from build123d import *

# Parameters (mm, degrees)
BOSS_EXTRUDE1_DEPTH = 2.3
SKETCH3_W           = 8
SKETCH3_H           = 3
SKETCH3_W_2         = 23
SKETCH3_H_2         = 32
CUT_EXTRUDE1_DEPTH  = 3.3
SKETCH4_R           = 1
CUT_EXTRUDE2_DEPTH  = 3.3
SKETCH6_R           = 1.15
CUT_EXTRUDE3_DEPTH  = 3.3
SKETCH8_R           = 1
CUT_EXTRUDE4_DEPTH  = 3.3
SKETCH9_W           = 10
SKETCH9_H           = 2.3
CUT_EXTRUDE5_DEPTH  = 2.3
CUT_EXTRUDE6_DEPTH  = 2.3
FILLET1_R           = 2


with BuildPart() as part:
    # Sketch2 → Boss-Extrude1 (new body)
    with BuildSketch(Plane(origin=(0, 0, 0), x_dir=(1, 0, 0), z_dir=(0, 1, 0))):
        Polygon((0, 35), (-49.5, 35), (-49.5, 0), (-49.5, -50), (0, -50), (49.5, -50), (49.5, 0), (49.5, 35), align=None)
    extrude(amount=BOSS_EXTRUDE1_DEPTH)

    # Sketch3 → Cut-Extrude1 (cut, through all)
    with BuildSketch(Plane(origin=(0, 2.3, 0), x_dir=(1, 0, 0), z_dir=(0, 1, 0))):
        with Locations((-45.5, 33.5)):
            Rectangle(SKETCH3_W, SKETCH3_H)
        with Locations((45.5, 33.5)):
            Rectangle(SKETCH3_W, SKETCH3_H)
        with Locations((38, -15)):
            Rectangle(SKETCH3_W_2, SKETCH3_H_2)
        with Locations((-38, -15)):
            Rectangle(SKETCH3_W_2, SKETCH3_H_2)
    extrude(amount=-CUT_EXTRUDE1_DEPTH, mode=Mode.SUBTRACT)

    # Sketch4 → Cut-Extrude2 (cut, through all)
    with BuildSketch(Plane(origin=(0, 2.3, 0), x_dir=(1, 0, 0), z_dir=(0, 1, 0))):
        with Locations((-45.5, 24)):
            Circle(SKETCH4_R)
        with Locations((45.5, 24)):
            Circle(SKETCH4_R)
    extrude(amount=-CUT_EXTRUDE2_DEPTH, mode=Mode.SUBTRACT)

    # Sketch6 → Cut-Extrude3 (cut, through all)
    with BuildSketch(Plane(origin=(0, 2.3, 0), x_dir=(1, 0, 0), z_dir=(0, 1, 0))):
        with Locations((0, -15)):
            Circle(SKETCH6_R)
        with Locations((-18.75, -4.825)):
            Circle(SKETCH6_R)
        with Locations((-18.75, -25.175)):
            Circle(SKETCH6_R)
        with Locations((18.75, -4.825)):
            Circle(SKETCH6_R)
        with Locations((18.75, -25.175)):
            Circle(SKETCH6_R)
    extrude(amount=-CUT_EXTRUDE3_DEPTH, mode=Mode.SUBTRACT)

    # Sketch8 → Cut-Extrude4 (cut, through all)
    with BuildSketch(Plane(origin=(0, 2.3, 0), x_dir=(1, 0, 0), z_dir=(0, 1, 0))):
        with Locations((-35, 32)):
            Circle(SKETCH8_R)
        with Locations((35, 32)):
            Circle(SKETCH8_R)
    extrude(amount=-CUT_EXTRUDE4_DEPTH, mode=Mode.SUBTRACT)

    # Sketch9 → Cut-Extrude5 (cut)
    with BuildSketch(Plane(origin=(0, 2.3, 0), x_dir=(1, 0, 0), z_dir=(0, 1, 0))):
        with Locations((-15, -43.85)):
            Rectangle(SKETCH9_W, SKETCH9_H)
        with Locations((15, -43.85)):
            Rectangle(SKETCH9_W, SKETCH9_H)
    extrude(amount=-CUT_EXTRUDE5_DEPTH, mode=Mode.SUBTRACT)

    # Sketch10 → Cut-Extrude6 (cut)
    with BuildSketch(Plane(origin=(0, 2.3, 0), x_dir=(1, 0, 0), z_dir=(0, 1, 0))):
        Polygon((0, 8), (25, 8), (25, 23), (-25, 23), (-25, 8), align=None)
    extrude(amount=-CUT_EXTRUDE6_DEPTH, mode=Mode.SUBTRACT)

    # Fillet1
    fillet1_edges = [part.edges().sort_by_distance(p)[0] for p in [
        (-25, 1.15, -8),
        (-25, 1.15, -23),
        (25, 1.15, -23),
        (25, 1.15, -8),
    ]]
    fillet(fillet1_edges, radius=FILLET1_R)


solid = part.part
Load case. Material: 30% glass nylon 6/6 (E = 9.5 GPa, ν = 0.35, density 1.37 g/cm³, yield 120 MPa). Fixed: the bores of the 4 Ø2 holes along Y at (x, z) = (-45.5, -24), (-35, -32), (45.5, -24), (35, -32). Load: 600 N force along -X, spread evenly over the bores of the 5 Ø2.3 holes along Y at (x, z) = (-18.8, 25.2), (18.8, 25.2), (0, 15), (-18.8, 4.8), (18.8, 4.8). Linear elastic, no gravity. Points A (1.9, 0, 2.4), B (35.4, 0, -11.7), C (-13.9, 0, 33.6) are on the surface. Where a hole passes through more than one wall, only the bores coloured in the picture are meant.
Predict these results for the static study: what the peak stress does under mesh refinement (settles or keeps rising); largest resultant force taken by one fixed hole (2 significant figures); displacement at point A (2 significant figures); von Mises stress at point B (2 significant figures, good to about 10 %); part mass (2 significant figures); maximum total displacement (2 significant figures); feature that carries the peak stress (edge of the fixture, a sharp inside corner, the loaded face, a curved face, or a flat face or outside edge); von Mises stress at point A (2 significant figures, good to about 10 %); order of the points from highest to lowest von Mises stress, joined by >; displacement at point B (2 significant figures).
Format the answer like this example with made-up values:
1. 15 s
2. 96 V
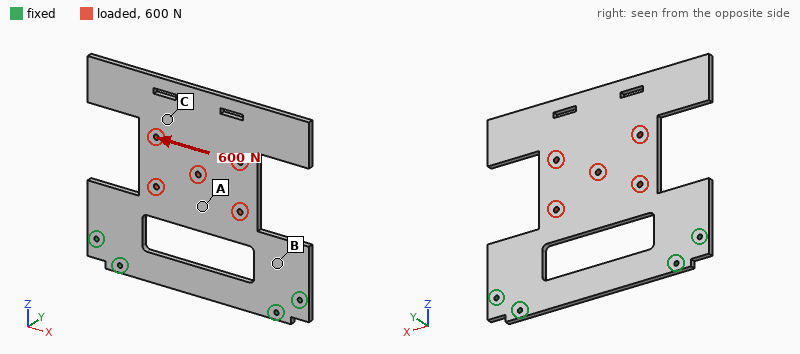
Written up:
1. keeps rising
2. 390 N
3. 0.084 mm
4. 13 MPa
5. 19 g
6. 0.12 mm
7. edge of the fixture
8. 6.0 MPa
9. B > A > C
10. 0.040 mm
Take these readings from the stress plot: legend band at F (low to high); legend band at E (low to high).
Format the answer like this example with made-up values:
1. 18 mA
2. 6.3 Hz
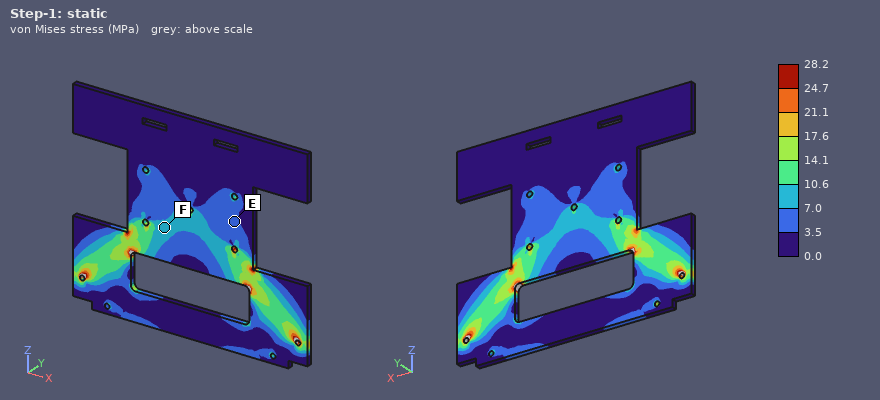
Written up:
1. 7.0 to 10.6 MPa
2. 3.5 to 7.0 MPa
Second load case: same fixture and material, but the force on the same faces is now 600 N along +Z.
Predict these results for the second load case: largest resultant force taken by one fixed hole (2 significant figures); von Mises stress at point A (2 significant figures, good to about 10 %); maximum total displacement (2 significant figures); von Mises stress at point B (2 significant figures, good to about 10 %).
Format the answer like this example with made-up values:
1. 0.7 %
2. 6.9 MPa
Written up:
1. 200 N
2. 2.5 MPa
3. 80 µm
4. 7.6 MPa
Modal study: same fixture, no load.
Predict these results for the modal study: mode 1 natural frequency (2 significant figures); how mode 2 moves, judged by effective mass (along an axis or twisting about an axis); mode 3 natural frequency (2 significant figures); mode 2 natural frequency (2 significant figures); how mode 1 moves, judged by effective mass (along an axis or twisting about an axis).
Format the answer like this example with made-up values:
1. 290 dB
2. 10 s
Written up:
1. 100 Hz
2. twisting about Z
3. 650 Hz
4. 270 Hz
5. along Y
